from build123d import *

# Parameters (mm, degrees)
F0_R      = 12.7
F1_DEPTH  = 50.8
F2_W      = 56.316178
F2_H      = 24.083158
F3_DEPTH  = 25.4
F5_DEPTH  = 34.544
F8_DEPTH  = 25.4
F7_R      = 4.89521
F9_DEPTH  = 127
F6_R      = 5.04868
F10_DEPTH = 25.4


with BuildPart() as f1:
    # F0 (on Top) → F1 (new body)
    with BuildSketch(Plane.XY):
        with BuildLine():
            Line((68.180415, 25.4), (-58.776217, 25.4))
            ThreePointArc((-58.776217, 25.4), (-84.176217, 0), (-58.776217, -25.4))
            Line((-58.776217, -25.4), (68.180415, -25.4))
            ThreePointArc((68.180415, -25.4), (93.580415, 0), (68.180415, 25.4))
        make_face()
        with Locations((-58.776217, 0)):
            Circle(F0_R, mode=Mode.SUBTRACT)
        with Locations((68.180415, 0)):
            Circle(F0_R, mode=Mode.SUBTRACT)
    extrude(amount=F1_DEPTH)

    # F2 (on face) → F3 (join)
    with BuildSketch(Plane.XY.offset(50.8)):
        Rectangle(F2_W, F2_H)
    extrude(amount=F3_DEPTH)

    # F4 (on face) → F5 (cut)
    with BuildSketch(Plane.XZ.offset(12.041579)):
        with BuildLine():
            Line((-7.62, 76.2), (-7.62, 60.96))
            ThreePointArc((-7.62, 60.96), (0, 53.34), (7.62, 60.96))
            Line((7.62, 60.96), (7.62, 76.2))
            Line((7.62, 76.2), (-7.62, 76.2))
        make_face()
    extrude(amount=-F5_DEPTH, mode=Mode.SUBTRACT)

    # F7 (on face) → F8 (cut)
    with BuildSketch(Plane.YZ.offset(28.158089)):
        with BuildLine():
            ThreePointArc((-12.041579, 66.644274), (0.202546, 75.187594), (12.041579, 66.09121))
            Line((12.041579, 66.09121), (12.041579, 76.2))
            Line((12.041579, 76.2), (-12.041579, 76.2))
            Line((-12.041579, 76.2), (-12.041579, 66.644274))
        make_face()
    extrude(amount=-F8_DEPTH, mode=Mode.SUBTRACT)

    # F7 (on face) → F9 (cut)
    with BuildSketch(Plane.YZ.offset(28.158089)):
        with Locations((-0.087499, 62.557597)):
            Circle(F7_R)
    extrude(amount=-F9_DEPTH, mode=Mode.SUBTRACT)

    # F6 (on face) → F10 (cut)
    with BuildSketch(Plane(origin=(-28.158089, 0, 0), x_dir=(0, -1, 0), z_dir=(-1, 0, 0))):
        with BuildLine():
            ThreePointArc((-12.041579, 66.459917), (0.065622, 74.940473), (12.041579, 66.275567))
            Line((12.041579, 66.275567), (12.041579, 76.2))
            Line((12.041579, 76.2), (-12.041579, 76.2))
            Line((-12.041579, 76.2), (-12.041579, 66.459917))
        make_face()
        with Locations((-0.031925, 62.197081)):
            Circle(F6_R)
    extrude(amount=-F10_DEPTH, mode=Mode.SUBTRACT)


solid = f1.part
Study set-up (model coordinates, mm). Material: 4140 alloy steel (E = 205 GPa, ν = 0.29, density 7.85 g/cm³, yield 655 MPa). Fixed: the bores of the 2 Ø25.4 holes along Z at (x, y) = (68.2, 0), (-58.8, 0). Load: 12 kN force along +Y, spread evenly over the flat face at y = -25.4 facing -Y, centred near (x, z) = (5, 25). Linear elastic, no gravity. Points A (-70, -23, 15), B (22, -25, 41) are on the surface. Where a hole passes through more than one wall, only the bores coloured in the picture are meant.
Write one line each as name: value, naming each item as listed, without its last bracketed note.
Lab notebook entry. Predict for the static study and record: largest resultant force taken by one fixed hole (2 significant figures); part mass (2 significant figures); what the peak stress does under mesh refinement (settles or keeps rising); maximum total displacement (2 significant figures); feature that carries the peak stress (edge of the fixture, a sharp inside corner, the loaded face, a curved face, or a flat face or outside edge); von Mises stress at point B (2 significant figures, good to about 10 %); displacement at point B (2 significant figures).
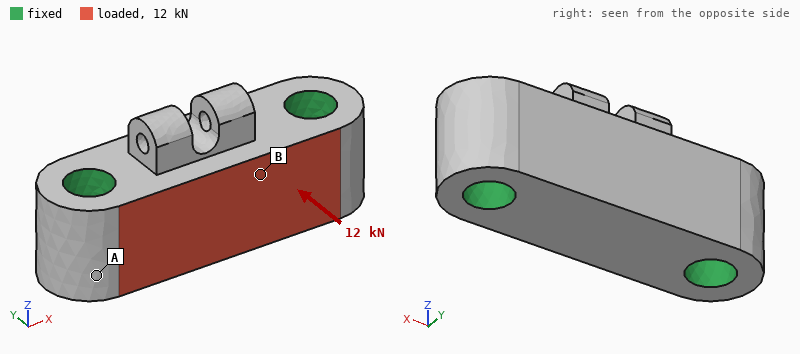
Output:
largest resultant force taken by one fixed hole: 6.0 kN
part mass: 3.1 kg
what the peak stress does under mesh refinement: keeps rising
maximum total displacement: 1.5 µm
feature that carries the peak stress: edge of the fixture
von Mises stress at point B: 2.9 MPa
displacement at point B: 1.3 µm
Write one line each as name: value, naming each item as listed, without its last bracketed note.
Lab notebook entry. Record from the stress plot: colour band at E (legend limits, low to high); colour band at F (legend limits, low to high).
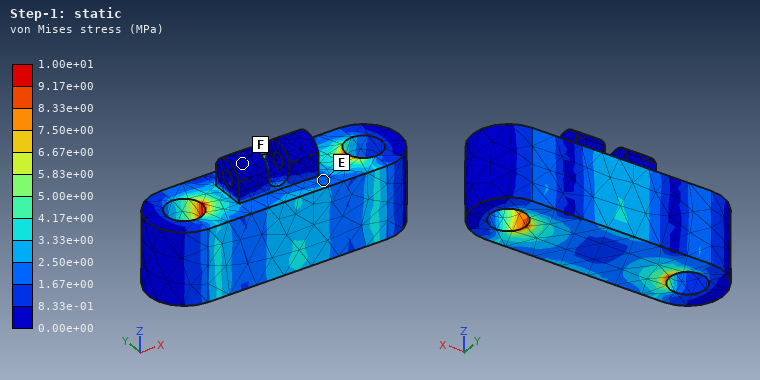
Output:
colour band at E: 1.67e+00 to 2.50e+00 MPa
colour band at F: 0.00e+00 to 8.33e-01 MPa
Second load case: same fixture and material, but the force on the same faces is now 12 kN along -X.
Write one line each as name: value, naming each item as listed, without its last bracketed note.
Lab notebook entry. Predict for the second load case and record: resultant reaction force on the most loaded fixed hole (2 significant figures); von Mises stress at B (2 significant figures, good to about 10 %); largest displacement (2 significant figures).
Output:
resultant reaction force on the most loaded fixed hole: 6.3 kN
von Mises stress at B: 3.4 MPa
largest displacement: 0.70 µm
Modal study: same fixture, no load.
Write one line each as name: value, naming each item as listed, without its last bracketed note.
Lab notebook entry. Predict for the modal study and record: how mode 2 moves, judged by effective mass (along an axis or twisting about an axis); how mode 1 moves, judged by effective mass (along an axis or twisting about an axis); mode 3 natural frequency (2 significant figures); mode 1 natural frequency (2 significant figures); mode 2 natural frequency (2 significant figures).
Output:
how mode 2 moves, judged by effective mass: along Z
how mode 1 moves, judged by effective mass: along Y
mode 3 natural frequency: 12 kHz
mode 1 natural frequency: 9300 Hz
mode 2 natural frequency: 11 kHz
